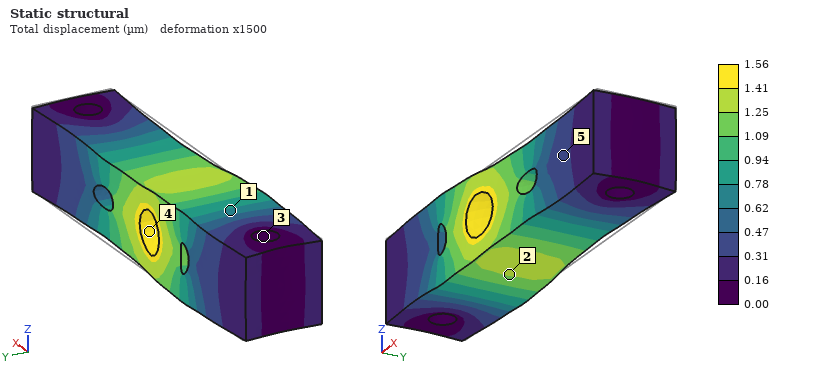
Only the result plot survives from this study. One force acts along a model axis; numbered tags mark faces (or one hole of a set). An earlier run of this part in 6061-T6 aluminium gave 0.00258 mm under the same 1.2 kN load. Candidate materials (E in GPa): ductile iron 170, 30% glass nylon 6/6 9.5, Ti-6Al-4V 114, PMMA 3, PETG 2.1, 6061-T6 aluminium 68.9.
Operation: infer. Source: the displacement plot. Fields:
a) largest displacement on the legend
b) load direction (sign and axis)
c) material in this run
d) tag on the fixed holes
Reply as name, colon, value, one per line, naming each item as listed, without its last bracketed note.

largest displacement on the legend: 1.56 µm
load direction: -X
material in this run: Ti-6Al-4V
tag on the fixed holes: 3
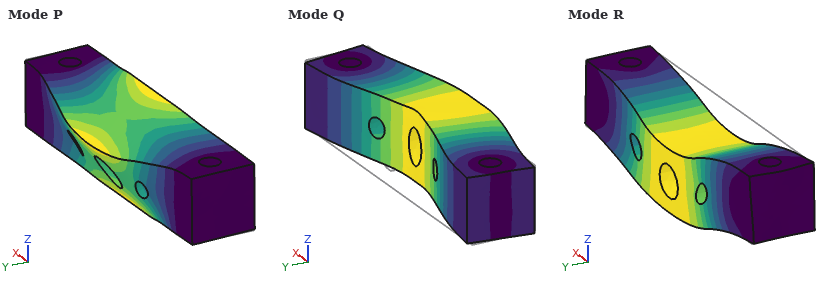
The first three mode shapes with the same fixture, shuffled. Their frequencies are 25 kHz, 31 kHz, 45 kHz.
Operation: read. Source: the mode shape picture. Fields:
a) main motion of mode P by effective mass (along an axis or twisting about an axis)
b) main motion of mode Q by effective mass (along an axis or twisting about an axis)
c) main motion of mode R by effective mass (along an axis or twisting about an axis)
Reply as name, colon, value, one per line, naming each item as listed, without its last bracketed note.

main motion of mode P by effective mass: twisting about X
main motion of mode Q by effective mass: along Y
main motion of mode R by effective mass: along Z
